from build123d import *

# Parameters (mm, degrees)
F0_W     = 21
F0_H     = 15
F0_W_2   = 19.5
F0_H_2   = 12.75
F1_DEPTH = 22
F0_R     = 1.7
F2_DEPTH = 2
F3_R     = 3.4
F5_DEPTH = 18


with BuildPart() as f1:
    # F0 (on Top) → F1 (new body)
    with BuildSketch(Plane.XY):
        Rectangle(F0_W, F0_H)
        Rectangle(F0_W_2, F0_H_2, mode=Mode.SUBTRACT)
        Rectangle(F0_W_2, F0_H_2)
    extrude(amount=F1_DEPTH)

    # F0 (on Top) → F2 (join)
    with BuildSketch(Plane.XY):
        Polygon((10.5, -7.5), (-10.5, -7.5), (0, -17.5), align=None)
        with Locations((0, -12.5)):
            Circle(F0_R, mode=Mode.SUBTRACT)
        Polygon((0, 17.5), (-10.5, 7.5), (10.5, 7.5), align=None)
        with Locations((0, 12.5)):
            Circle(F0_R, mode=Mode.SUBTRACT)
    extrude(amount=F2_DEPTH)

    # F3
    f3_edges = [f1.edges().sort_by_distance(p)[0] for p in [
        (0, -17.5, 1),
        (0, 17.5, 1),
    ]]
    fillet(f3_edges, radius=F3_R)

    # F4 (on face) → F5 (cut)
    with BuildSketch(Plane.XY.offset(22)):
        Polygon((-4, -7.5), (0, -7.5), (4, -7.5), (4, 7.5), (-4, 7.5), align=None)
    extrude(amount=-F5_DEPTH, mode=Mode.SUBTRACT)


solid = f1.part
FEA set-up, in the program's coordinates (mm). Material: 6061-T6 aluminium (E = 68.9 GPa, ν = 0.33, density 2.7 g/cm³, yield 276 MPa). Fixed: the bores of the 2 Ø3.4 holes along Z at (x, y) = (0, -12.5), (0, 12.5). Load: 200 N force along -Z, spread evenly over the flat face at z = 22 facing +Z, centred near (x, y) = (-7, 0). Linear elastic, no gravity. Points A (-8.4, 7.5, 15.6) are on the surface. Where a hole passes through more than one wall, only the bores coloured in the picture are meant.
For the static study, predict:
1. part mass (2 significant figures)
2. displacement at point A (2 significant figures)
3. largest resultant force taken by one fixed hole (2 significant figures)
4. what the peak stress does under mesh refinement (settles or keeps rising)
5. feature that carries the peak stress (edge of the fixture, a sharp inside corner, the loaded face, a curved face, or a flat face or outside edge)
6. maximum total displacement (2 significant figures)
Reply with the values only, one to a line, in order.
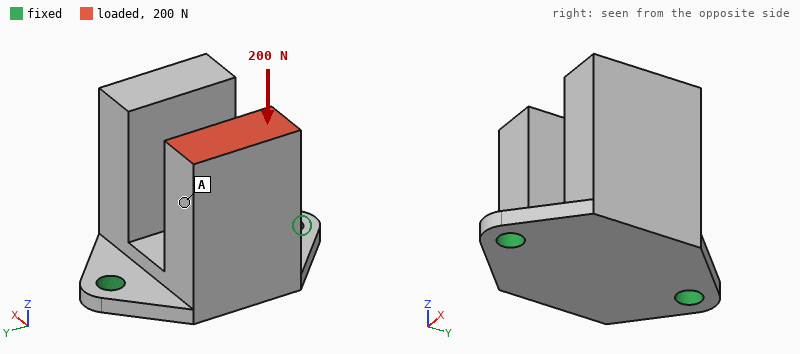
14 g
52 µm
120 N
keeps rising
edge of the fixture
72 µm
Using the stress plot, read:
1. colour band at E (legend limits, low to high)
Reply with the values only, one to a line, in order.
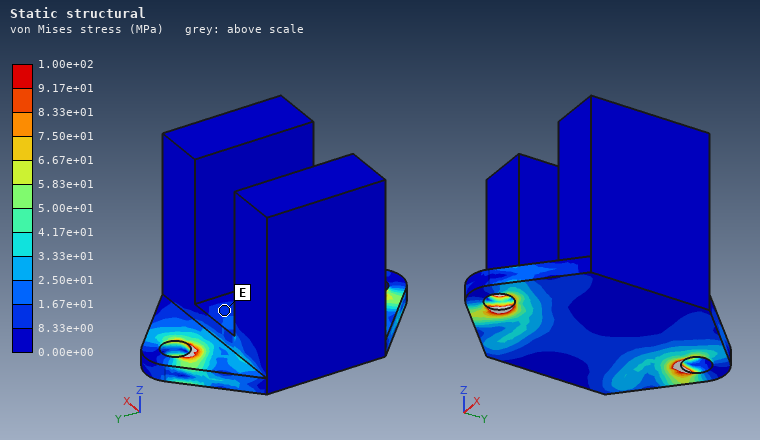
8.33e+00 to 1.67e+01 MPa
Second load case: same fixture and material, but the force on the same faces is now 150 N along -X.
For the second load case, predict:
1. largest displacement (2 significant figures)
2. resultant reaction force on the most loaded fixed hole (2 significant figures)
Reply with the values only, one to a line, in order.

0.19 mm
97 N
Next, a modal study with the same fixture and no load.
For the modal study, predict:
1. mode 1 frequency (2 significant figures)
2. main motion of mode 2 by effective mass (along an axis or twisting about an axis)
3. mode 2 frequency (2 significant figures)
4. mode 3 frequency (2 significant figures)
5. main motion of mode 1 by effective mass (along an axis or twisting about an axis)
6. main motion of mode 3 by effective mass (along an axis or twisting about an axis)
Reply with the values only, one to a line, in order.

2400 Hz
along Z
5500 Hz
7400 Hz
along X
along Y
